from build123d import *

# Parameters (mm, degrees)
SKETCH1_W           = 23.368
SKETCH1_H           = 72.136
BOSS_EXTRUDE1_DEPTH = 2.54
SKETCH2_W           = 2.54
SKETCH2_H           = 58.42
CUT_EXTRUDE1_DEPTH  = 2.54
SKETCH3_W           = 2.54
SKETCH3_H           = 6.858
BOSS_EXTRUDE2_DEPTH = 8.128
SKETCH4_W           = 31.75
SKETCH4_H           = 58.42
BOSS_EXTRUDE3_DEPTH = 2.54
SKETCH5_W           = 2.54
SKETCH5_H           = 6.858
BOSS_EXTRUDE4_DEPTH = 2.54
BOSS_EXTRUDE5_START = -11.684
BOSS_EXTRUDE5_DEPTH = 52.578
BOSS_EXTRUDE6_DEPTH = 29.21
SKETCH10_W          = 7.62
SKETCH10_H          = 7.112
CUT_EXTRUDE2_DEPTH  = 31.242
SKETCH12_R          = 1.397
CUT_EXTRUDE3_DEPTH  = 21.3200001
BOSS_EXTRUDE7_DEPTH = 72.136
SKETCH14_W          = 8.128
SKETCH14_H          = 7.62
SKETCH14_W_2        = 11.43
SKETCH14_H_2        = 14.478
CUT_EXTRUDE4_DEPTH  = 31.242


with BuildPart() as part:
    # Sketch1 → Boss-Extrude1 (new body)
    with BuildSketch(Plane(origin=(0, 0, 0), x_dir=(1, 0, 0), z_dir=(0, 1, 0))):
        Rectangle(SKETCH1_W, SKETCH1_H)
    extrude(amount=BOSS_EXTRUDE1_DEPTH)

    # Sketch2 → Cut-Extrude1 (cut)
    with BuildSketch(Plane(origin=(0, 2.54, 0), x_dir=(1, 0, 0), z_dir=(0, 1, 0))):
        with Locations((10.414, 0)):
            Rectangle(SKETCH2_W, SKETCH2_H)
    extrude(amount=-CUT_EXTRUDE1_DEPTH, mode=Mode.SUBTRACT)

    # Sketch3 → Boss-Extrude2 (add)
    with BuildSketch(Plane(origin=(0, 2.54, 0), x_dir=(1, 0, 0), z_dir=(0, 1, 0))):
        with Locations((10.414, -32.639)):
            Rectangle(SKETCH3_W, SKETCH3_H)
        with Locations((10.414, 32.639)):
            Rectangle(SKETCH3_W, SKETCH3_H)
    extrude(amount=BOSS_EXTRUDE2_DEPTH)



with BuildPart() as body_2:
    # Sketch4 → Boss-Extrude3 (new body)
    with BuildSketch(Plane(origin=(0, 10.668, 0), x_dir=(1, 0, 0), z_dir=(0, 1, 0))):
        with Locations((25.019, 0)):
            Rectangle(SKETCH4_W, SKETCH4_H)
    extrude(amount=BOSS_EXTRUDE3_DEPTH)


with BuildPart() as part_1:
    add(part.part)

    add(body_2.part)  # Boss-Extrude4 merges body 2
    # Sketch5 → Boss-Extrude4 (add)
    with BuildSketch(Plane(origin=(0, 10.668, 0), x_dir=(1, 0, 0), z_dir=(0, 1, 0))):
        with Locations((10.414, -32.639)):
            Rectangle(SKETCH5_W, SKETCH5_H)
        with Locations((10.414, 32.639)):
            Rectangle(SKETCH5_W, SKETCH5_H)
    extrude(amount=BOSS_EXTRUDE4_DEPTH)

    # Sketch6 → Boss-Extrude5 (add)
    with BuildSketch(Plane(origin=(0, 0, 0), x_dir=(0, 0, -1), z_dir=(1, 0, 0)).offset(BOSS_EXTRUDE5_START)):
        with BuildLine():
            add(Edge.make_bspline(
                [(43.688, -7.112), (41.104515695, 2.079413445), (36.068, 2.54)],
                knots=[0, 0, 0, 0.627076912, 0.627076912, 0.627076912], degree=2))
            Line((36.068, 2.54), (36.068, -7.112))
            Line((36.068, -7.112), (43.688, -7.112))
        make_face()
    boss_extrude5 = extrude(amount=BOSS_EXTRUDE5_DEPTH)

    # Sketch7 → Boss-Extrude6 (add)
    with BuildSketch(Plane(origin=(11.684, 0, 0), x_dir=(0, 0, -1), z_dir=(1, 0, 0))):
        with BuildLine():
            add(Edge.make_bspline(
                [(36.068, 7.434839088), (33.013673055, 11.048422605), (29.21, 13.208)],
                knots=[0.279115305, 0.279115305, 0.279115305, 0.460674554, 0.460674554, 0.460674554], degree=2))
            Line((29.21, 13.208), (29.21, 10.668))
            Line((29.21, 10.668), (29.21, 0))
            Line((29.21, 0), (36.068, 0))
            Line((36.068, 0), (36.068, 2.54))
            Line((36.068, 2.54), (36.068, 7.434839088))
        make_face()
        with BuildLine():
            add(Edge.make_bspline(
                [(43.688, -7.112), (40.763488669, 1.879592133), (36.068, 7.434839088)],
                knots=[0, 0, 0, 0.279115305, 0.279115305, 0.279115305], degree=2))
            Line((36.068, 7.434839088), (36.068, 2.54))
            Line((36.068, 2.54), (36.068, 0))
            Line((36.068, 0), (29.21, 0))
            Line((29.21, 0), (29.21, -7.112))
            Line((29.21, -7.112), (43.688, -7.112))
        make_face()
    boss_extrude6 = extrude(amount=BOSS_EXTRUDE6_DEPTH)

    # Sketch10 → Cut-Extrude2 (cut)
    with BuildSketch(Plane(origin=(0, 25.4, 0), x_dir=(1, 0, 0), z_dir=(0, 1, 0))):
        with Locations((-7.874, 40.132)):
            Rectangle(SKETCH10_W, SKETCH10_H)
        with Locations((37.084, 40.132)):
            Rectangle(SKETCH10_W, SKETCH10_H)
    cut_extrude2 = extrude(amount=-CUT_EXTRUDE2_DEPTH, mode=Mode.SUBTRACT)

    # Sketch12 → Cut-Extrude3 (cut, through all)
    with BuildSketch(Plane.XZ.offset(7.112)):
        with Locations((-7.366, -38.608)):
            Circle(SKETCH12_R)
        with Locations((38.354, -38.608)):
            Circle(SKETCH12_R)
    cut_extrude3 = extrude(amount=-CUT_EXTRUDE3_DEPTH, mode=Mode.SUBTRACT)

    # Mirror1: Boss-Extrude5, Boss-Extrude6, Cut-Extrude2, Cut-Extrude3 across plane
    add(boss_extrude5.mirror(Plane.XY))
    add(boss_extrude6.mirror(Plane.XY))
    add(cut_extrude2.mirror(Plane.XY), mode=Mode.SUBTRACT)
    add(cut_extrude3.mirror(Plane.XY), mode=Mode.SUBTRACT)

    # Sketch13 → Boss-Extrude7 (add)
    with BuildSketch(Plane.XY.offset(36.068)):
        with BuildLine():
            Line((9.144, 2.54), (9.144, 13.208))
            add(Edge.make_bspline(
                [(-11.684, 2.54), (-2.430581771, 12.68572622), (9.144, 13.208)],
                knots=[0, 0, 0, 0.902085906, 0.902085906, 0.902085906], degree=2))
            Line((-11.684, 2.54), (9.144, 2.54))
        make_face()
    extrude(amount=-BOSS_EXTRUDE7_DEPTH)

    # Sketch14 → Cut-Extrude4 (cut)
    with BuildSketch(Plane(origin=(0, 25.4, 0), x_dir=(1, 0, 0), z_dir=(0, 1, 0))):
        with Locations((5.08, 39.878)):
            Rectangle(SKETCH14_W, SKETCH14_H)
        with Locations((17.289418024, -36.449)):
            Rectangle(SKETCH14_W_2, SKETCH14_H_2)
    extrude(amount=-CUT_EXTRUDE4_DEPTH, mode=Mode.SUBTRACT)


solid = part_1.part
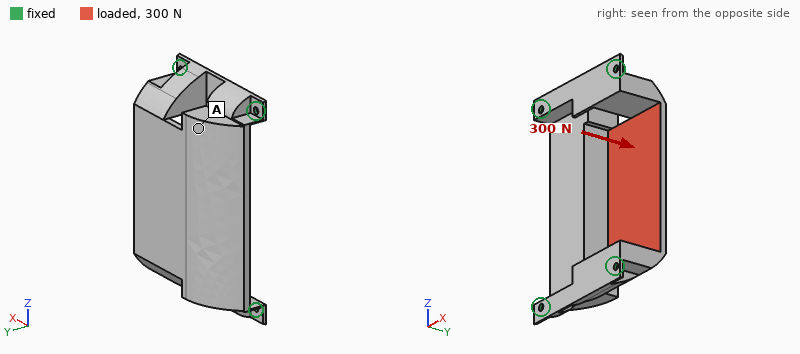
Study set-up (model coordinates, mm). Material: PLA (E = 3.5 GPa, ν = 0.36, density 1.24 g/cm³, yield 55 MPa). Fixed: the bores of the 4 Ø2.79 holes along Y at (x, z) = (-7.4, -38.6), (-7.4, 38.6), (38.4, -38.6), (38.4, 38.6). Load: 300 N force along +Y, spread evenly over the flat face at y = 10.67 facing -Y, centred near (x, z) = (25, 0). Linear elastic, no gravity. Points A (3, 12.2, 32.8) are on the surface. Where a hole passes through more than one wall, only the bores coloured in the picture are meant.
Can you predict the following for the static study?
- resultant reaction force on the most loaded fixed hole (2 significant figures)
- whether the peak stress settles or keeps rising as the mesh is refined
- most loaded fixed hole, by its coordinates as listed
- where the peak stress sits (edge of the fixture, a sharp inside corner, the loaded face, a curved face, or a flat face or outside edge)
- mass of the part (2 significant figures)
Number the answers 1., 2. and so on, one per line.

1. 150 N
2. keeps rising
3. (38.4, -38.6)
4. edge of the fixture
5. 36 g
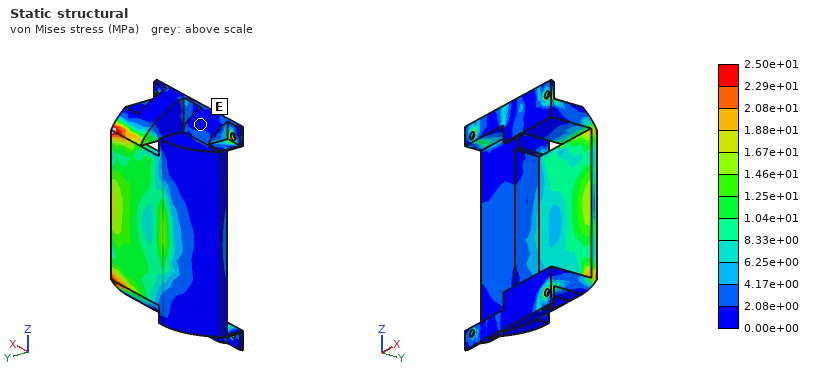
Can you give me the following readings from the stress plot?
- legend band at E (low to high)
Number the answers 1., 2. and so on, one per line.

1. 0.00e+00 to 2.08e+00 MPa
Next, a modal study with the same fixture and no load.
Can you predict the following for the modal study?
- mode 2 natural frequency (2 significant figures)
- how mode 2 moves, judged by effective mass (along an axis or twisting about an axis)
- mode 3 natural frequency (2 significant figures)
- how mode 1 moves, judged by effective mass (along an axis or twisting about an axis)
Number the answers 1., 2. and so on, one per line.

1. 1400 Hz
2. along Y
3. 1600 Hz
4. along Z
